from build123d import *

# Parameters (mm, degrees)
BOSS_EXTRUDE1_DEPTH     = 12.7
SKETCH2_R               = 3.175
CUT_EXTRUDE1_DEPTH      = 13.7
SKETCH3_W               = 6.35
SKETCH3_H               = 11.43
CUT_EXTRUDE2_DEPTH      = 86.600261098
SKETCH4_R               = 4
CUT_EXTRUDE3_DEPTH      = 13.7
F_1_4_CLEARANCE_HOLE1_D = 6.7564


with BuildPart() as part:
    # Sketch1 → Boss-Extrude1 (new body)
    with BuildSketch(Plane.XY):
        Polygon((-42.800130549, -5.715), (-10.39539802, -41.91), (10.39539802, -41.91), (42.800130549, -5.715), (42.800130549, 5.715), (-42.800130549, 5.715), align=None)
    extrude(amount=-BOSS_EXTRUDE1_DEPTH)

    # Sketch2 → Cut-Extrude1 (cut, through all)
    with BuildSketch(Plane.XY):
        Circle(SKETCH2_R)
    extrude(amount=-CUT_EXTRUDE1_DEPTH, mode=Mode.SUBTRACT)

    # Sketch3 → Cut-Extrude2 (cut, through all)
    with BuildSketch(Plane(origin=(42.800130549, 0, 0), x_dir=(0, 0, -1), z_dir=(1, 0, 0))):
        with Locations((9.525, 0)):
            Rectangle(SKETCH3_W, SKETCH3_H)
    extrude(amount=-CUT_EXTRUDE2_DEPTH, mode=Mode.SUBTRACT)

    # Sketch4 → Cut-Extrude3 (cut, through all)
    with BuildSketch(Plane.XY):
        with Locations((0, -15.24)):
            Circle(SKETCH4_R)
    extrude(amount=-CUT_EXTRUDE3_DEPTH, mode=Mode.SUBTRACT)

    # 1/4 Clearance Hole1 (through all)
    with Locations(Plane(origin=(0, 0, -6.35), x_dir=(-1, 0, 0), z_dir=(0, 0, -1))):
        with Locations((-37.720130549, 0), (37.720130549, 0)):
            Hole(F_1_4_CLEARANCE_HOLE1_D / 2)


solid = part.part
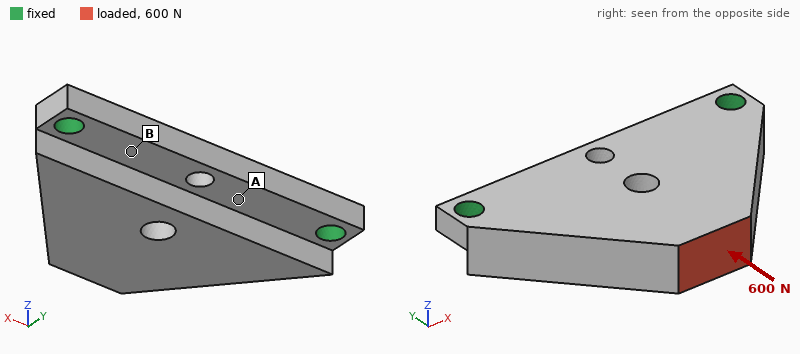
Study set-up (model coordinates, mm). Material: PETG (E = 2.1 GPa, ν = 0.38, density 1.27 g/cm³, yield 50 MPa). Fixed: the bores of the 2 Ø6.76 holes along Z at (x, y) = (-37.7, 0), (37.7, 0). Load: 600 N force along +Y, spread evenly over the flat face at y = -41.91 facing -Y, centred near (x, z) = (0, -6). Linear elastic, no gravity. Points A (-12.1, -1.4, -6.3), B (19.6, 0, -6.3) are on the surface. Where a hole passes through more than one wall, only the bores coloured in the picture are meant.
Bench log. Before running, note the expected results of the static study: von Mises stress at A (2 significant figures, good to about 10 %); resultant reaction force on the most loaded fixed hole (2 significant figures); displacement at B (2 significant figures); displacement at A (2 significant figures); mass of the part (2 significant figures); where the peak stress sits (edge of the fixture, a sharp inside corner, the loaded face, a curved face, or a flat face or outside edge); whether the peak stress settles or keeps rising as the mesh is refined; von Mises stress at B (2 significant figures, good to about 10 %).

1.1 MPa
360 N
0.068 mm
0.081 mm
37 g
edge of the fixture
keeps rising
2.4 MPa
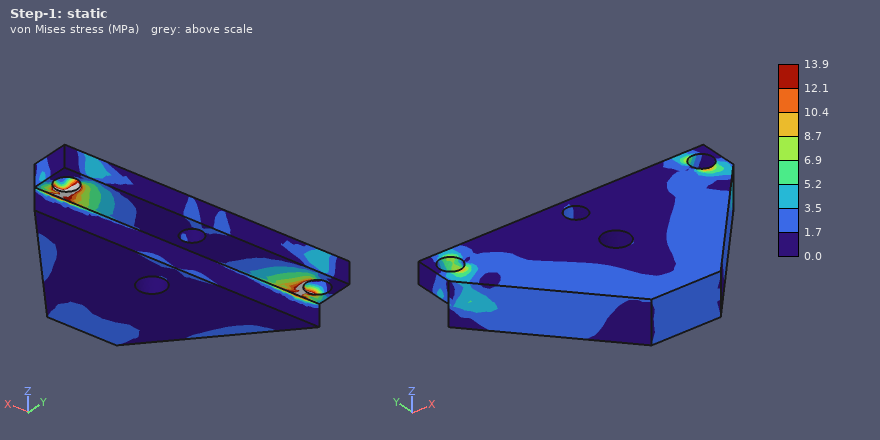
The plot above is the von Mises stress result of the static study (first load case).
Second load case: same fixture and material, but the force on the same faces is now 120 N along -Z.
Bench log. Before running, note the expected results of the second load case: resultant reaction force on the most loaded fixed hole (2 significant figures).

73 N
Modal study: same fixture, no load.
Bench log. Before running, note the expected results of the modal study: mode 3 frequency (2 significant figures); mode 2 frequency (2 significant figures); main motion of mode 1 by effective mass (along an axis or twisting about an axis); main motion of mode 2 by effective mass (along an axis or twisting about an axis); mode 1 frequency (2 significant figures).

2800 Hz
2100 Hz
along Z
along Z
600 Hz
